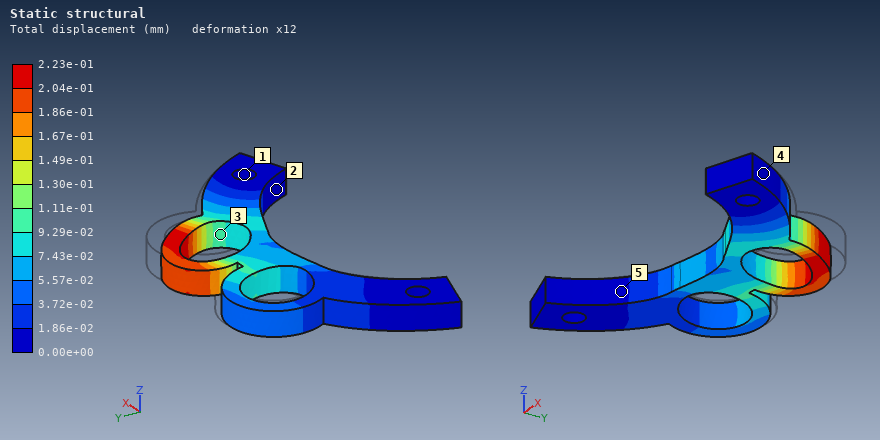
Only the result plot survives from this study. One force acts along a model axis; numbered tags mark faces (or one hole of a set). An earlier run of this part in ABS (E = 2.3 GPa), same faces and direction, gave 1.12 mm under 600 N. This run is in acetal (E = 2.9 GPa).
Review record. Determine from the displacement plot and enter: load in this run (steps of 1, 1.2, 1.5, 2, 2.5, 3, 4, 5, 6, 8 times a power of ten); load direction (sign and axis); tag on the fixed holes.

150 N
-X
1
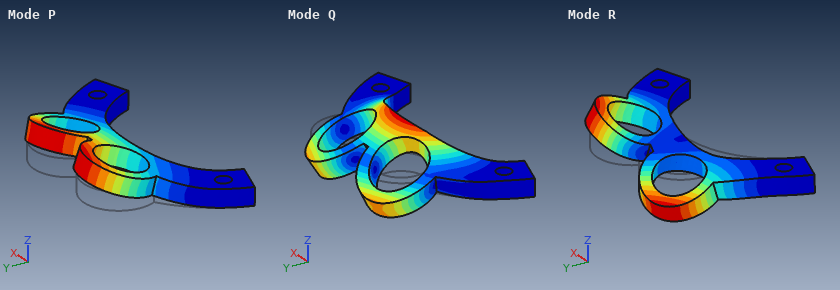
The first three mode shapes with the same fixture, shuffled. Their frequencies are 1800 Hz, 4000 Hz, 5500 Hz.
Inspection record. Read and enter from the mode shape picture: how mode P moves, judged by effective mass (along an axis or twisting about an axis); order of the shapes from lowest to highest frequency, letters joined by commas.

along Z
P, R, Q
